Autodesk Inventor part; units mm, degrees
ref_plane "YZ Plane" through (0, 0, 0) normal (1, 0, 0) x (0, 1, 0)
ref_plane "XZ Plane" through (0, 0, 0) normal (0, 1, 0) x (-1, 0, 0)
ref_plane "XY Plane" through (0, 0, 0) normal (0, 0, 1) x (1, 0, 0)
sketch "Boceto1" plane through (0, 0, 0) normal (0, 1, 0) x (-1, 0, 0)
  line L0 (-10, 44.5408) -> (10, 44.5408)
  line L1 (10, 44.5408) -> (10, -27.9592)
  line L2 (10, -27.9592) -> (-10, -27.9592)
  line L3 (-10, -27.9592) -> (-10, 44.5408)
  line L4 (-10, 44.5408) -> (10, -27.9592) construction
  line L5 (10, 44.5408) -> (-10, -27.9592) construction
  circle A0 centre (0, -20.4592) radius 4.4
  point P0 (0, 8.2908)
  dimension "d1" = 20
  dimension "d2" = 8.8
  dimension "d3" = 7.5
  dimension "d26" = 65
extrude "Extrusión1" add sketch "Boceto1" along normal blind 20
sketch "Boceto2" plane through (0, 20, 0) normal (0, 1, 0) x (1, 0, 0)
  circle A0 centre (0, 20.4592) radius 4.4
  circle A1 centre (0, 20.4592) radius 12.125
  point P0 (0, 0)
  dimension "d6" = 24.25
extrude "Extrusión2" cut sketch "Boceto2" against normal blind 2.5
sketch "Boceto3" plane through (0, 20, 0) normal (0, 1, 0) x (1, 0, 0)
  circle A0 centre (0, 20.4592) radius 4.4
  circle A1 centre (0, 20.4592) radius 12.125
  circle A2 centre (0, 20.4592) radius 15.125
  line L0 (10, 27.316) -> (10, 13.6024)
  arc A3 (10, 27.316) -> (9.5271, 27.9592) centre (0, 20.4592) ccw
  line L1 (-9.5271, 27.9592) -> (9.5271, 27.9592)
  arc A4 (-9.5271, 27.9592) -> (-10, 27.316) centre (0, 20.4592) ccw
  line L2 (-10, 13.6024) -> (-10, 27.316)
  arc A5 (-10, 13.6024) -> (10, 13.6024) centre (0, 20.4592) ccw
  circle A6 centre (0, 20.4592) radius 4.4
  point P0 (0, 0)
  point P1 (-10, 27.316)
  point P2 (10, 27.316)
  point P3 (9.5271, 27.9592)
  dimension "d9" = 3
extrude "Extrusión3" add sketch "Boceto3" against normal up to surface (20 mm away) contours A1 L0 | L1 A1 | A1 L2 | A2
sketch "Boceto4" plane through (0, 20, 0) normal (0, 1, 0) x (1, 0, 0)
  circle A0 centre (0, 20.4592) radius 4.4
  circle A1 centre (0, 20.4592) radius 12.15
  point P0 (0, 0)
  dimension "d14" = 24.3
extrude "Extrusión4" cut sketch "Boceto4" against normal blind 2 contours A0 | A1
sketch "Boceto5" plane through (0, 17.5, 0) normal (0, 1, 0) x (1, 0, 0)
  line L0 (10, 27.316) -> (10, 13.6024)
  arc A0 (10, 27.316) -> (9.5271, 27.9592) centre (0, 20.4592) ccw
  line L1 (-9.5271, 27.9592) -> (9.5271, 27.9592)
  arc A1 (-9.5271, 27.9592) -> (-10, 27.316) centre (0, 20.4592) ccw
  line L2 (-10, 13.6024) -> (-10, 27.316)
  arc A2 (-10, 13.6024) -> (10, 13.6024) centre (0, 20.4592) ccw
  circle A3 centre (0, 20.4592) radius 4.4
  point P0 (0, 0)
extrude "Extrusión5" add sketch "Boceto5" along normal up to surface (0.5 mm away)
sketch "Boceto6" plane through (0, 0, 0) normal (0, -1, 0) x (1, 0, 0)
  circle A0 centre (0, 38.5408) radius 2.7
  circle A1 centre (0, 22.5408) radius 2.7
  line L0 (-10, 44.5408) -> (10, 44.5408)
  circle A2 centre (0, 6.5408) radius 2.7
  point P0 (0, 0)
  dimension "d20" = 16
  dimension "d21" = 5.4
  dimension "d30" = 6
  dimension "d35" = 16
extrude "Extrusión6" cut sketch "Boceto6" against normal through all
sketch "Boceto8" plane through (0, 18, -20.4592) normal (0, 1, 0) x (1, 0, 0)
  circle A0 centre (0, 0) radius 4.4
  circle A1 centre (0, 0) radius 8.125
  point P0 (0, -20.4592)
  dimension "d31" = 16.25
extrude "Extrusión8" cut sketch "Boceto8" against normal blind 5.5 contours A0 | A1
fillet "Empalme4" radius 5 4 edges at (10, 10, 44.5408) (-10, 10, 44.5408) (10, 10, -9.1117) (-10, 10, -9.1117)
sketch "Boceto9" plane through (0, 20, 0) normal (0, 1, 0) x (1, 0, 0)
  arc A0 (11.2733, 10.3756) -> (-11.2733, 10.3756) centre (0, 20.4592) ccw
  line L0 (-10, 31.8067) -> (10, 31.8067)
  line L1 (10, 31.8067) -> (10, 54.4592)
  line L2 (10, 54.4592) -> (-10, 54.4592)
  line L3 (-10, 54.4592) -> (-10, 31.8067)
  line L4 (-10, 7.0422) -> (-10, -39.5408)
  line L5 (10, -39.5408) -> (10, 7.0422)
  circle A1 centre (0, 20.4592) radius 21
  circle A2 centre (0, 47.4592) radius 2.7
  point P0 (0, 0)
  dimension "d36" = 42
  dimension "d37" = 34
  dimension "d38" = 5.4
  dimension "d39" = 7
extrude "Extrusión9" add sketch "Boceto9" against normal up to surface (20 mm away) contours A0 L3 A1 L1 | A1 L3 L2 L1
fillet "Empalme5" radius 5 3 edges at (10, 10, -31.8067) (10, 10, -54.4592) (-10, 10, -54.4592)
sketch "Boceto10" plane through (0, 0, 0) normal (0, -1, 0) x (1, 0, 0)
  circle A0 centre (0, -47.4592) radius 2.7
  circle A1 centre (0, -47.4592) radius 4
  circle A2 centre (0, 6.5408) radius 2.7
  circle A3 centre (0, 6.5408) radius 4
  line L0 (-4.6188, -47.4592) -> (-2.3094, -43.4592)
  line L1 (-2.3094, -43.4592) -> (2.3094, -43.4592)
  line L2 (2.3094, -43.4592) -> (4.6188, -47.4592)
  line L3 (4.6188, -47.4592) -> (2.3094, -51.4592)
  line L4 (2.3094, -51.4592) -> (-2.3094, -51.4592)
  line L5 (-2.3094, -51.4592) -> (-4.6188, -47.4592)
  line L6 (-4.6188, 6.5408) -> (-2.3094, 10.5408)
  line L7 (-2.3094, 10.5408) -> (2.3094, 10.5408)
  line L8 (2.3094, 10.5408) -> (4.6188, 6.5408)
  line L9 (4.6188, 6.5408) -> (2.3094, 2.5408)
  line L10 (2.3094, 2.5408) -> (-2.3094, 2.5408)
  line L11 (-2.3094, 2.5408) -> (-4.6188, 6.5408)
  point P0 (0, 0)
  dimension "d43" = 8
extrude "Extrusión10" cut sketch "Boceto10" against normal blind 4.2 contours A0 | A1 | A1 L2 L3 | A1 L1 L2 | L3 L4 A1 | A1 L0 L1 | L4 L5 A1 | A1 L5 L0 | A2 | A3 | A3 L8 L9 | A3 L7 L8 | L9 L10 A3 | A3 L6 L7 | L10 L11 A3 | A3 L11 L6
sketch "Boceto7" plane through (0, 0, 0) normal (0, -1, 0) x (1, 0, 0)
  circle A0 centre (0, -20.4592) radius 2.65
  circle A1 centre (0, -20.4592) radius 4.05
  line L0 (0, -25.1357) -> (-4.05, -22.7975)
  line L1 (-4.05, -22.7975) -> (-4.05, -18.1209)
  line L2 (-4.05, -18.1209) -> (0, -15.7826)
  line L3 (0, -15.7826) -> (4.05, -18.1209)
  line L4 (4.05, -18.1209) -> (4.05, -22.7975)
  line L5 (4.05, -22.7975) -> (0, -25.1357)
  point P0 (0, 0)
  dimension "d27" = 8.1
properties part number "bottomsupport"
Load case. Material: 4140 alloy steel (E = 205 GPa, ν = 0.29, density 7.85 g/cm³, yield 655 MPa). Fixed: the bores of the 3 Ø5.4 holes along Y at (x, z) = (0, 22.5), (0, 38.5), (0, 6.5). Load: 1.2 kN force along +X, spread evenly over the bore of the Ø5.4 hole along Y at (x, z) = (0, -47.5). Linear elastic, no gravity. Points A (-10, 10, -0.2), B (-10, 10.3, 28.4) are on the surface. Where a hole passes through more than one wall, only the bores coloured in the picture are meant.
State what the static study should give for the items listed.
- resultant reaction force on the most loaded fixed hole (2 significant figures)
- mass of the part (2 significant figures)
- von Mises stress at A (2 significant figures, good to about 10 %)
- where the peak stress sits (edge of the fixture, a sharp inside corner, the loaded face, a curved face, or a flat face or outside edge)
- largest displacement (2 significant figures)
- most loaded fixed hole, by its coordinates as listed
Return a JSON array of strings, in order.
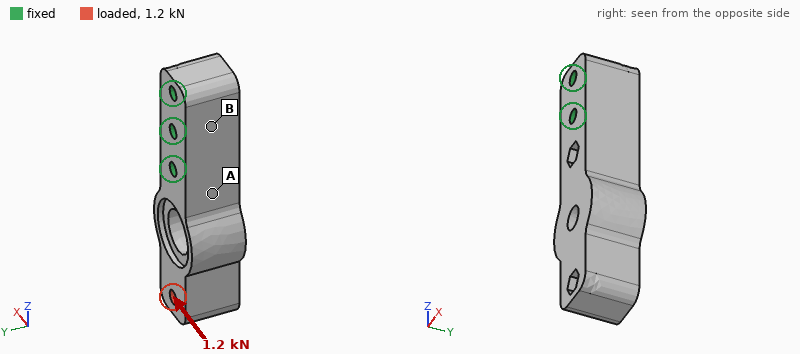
["3.3 kN", "290 g", "45 MPa", "edge of the fixture", "41 µm", "(0, 6.5)"]
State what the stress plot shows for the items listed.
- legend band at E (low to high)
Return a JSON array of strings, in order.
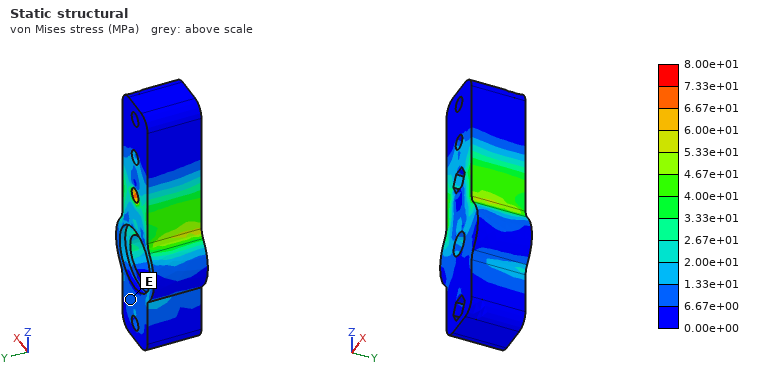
["6.67e+00 to 1.33e+01 MPa"]
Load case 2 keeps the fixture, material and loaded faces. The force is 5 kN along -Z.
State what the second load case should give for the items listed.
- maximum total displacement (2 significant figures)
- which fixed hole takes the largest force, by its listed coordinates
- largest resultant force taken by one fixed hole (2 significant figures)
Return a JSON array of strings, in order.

["19 µm", "(0, 6.5)", "4.1 kN"]
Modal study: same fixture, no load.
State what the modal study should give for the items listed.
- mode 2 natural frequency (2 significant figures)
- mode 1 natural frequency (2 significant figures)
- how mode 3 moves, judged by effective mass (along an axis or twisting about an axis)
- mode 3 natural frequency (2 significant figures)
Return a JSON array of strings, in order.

["3500 Hz", "3500 Hz", "twisting about Z", "10 kHz"]
